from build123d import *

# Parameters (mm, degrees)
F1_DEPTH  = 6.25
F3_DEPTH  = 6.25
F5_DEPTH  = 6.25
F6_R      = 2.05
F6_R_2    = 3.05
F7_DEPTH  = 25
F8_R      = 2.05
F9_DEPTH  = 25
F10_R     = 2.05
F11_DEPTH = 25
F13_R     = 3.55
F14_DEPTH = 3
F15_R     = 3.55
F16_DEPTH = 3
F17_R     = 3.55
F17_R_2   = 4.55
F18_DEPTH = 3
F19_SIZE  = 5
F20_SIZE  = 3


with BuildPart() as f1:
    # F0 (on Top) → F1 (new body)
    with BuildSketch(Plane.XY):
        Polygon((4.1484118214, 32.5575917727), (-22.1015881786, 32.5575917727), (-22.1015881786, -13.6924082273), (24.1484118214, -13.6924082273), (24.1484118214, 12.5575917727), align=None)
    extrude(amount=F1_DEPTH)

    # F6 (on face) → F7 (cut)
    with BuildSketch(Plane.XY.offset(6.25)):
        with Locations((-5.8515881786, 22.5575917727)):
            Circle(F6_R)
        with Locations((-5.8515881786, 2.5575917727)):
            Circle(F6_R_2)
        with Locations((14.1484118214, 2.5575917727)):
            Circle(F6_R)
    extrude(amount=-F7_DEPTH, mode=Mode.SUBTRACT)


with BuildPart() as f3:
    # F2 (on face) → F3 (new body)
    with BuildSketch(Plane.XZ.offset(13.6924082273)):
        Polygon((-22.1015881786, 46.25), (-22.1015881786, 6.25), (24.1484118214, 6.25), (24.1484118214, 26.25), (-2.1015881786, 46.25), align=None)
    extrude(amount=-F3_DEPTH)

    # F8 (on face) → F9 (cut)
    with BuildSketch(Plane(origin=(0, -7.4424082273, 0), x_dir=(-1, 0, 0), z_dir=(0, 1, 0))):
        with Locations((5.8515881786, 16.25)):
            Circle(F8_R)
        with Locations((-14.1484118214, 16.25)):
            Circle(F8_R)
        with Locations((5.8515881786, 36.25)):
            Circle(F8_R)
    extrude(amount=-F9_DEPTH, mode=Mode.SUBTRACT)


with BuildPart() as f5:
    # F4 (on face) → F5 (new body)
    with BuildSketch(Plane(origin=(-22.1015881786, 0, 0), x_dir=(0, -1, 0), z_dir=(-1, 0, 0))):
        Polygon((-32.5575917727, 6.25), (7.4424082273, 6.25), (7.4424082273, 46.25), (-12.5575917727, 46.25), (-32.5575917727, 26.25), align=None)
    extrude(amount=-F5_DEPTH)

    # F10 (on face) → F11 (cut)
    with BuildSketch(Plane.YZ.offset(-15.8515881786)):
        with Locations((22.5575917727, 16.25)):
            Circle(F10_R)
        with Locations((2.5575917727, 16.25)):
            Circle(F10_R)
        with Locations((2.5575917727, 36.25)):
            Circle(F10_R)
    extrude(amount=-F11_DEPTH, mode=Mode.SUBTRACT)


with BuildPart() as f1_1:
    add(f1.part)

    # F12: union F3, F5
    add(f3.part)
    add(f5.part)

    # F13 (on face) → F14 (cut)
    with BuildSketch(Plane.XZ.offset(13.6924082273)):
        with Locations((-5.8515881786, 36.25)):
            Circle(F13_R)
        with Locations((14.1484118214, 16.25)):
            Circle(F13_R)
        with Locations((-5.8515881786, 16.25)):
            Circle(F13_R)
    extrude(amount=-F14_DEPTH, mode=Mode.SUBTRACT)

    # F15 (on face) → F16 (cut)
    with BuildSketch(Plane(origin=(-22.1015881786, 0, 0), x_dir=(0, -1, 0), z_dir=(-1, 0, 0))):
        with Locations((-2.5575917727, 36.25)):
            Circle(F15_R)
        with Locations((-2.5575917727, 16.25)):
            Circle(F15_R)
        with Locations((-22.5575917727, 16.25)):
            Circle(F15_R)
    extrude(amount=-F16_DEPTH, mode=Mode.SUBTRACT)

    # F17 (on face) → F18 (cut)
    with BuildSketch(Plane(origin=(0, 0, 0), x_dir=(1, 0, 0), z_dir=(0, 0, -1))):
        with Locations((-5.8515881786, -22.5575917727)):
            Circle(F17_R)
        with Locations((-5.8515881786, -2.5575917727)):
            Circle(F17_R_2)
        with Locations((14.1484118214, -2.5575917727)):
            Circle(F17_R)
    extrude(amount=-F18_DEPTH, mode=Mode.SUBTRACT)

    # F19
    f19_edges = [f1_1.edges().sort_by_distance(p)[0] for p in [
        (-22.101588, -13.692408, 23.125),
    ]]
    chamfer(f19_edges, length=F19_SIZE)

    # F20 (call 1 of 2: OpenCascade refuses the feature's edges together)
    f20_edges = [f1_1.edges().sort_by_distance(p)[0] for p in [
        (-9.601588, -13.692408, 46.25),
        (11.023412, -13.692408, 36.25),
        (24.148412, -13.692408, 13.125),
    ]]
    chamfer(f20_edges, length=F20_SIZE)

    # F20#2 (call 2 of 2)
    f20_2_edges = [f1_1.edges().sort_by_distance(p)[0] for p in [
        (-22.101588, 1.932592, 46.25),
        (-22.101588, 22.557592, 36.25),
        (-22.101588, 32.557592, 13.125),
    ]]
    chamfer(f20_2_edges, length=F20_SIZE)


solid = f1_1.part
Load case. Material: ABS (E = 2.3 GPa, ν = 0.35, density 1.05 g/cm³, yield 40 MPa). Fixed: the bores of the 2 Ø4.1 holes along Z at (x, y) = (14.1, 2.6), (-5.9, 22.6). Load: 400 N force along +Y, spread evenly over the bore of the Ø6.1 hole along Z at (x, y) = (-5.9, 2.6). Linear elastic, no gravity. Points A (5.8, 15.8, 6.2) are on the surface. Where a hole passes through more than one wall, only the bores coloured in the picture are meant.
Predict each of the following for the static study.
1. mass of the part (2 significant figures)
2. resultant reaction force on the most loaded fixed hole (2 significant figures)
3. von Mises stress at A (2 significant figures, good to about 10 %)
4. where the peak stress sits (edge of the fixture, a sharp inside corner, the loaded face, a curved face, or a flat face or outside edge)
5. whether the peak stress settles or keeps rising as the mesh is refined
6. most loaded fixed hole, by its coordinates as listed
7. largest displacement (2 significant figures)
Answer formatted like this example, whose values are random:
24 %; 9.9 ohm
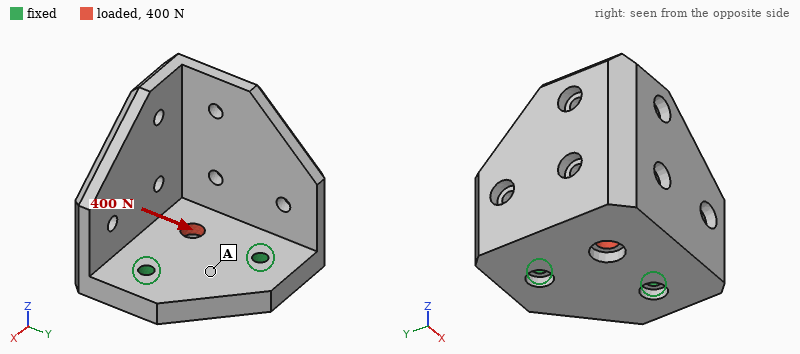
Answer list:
29 g; 320 N; 1.5 MPa; edge of the fixture; keeps rising; (-5.9, 22.6); 73 µm
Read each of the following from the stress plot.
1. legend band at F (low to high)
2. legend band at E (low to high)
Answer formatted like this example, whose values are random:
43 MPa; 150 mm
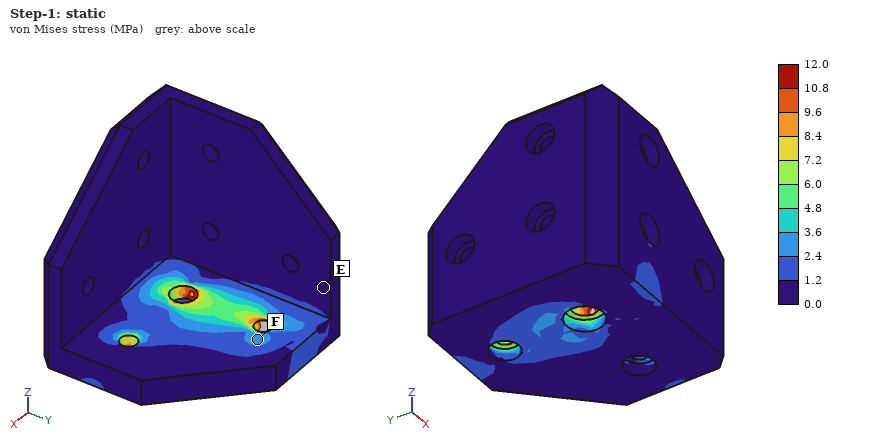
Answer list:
2.4 to 3.6 MPa; 0.0 to 1.2 MPa
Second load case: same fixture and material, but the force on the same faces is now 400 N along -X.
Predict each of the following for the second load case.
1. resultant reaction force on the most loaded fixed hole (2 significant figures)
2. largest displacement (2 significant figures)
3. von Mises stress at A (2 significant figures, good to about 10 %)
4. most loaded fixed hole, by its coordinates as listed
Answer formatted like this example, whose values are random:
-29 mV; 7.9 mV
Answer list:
320 N; 73 µm; 1.3 MPa; (14.1, 2.6)
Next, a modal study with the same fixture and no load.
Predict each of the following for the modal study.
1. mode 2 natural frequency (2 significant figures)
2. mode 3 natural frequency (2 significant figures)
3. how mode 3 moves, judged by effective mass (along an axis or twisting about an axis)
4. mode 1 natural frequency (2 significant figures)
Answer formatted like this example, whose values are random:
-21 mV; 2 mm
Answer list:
940 Hz; 1800 Hz; along Z; 400 Hz
